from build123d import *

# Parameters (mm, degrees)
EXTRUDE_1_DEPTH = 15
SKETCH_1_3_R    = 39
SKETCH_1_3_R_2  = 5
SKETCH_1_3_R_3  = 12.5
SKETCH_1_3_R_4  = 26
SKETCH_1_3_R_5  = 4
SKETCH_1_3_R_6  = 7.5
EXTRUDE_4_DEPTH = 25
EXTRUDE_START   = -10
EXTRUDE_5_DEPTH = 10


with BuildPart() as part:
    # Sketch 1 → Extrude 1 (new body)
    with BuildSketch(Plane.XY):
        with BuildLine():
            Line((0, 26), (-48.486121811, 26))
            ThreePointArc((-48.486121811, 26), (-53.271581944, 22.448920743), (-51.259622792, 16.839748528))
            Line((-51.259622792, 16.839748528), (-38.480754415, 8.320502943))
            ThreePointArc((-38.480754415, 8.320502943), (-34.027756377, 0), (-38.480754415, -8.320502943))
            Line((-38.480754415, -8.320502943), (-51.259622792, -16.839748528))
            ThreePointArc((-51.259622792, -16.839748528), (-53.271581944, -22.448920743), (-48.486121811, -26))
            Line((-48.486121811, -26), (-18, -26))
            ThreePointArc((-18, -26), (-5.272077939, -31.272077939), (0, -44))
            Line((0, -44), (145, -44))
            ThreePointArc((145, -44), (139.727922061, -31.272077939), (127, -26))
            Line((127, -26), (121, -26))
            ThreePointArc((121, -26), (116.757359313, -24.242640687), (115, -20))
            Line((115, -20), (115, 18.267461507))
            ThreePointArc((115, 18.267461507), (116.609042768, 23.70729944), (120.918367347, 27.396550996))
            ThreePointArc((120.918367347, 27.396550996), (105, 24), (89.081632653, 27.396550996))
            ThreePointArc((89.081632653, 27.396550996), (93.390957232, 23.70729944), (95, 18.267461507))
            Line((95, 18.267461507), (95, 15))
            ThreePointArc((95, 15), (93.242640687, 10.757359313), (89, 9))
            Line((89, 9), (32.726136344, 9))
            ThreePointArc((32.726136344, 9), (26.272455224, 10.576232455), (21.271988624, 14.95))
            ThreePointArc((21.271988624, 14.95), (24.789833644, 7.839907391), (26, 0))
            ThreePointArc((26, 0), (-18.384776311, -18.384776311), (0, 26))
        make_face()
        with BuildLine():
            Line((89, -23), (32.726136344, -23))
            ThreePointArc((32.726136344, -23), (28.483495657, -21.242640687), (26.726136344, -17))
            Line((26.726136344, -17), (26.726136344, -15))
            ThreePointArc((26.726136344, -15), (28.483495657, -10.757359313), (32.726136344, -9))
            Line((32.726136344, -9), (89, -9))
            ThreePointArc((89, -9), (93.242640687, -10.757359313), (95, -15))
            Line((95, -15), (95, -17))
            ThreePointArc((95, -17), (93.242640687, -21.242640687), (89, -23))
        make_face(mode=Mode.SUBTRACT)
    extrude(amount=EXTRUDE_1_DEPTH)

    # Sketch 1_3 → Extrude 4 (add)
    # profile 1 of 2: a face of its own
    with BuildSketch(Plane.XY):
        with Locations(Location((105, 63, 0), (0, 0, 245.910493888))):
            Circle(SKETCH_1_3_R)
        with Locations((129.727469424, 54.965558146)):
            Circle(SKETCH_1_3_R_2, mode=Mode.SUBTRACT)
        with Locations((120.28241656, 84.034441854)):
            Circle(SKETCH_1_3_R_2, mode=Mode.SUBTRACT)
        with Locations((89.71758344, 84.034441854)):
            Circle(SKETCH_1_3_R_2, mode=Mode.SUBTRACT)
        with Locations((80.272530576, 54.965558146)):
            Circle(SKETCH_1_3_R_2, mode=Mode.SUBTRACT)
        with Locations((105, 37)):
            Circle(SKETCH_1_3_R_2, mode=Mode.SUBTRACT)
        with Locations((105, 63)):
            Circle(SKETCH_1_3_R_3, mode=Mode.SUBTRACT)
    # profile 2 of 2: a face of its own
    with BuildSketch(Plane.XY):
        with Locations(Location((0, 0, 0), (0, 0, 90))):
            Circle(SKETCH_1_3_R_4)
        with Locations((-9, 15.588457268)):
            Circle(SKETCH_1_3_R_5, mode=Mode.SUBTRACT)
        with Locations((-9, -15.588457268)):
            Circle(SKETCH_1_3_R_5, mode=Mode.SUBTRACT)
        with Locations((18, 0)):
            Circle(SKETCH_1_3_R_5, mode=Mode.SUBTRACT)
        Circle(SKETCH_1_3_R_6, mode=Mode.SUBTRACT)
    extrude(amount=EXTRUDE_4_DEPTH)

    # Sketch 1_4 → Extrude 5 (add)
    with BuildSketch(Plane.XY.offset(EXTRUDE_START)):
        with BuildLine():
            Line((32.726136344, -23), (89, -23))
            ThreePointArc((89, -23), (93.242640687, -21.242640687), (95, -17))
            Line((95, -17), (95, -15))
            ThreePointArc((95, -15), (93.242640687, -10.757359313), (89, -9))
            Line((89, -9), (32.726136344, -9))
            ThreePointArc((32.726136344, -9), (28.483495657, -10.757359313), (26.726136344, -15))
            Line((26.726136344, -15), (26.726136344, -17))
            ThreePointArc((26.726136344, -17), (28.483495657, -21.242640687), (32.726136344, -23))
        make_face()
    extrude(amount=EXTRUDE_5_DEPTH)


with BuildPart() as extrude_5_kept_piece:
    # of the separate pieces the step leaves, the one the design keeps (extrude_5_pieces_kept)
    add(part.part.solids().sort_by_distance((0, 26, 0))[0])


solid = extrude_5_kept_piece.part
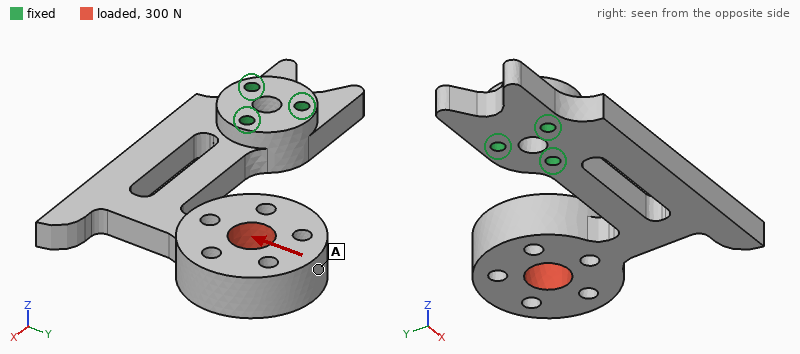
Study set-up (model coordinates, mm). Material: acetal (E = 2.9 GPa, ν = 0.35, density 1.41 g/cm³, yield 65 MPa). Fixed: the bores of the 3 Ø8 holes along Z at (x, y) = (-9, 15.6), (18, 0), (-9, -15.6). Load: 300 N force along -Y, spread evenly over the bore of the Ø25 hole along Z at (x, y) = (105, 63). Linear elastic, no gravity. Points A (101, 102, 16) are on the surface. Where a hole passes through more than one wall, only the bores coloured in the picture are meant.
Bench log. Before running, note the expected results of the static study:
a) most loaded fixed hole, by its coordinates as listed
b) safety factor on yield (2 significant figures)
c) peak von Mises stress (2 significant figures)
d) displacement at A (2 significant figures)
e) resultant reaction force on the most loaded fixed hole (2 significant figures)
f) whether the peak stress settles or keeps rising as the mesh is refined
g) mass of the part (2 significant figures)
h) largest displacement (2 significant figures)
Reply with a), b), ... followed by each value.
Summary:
a) (18, 0)
b) 7.2
c) 9.0 MPa
d) 0.98 mm
e) 770 N
f) settles
g) 340 g
h) 1.0 mm
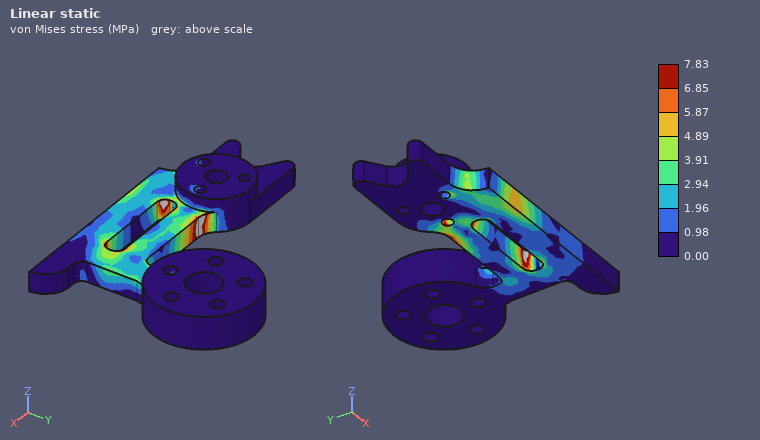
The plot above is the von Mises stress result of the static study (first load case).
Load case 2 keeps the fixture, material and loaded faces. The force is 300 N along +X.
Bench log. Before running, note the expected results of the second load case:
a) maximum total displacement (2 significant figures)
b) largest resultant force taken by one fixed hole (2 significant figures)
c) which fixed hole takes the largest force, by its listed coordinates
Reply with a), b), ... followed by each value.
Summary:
a) 2.2 mm
b) 700 N
c) (18, 0)
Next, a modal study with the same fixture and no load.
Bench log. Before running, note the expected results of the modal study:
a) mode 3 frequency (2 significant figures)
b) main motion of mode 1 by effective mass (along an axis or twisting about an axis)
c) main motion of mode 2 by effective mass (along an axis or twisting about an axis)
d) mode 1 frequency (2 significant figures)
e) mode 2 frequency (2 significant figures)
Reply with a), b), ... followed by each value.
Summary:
a) 210 Hz
b) along Z
c) along X
d) 79 Hz
e) 180 Hz
